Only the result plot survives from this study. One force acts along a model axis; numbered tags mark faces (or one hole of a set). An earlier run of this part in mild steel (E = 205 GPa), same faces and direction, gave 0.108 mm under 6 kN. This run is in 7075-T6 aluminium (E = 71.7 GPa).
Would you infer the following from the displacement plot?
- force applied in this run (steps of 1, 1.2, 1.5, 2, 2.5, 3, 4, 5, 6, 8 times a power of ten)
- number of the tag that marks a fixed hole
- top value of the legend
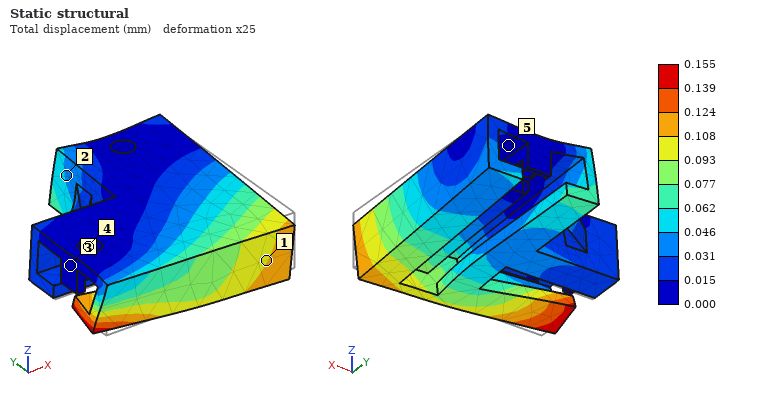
3 kN
4
0.155 mm
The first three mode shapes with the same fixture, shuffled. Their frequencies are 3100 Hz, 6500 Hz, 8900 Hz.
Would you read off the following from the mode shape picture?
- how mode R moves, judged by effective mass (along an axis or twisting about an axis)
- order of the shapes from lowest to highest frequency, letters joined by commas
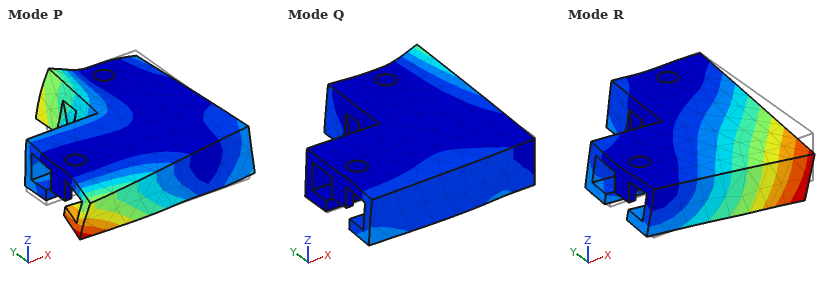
along Z
R, Q, P
